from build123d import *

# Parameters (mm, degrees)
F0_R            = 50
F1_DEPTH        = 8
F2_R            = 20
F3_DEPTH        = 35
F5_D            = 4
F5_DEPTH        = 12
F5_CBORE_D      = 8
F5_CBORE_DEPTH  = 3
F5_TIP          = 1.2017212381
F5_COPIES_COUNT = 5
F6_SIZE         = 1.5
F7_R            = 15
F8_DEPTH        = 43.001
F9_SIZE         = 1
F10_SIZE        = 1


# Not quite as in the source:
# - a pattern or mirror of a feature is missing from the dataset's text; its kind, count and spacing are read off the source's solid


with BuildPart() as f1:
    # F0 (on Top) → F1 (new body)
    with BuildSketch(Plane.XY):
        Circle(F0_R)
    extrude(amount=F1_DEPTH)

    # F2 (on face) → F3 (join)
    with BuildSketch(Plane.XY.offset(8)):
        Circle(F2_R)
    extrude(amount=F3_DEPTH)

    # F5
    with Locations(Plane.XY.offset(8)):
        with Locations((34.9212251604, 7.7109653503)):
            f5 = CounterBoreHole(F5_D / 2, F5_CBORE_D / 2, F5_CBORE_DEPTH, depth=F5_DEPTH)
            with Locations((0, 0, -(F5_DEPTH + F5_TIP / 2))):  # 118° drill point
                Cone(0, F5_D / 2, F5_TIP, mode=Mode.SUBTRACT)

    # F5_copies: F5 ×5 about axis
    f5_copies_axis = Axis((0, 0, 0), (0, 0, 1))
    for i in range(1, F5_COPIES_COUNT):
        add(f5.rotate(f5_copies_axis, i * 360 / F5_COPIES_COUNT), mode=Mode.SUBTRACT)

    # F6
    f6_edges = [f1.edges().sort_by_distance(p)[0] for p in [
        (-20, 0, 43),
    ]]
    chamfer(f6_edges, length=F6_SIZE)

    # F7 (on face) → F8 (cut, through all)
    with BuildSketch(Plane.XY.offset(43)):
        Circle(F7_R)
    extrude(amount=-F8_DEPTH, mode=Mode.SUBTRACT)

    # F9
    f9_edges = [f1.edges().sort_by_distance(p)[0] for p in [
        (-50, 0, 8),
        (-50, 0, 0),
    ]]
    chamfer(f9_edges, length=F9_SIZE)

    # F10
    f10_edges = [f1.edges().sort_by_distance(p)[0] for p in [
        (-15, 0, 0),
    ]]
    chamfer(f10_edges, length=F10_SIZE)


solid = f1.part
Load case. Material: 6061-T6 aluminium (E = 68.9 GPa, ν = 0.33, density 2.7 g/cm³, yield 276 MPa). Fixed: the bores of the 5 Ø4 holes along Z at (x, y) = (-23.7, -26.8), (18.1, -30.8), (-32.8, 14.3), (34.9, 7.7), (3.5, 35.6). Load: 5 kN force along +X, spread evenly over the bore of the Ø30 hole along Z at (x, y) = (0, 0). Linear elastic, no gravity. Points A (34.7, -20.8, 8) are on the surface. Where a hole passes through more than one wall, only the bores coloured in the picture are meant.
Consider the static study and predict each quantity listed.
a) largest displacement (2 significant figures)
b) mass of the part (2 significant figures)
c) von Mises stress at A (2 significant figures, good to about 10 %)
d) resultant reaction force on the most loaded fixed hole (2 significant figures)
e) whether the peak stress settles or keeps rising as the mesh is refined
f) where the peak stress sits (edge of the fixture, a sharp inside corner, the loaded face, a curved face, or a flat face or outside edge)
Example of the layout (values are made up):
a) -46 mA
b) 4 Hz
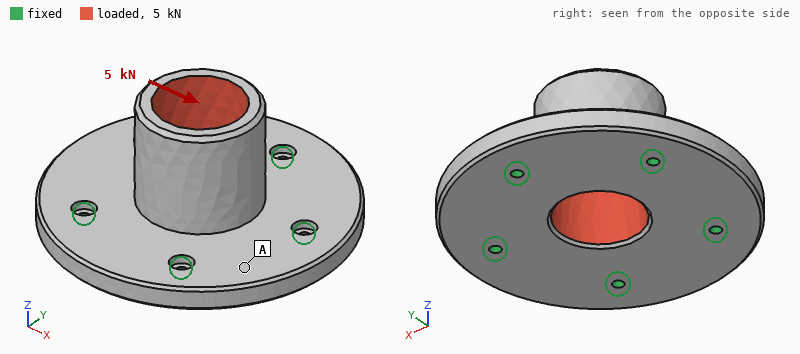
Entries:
a) 47 µm
b) 200 g
c) 5.5 MPa
d) 1.9 kN
e) keeps rising
f) edge of the fixture
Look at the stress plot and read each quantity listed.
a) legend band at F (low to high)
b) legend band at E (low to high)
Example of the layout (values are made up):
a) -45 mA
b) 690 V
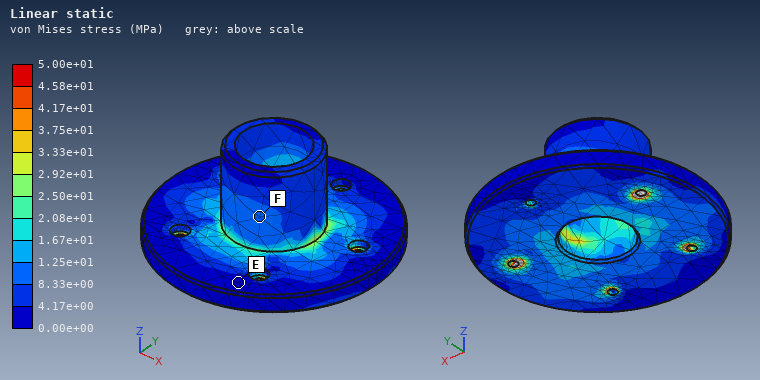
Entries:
a) 8.33e+00 to 1.25e+01 MPa
b) 0.00e+00 to 4.17e+00 MPa
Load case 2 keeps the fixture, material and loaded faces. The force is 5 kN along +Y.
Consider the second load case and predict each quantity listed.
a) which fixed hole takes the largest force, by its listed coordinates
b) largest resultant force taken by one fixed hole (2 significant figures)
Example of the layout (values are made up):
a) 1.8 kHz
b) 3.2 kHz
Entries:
a) (3.5, 35.6)
b) 1.9 kN
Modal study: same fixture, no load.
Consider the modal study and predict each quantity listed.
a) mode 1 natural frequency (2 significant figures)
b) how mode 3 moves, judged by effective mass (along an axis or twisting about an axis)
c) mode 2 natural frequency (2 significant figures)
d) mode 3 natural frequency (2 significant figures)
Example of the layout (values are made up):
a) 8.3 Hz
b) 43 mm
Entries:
a) 7200 Hz
b) along Z
c) 7200 Hz
d) 8200 Hz
